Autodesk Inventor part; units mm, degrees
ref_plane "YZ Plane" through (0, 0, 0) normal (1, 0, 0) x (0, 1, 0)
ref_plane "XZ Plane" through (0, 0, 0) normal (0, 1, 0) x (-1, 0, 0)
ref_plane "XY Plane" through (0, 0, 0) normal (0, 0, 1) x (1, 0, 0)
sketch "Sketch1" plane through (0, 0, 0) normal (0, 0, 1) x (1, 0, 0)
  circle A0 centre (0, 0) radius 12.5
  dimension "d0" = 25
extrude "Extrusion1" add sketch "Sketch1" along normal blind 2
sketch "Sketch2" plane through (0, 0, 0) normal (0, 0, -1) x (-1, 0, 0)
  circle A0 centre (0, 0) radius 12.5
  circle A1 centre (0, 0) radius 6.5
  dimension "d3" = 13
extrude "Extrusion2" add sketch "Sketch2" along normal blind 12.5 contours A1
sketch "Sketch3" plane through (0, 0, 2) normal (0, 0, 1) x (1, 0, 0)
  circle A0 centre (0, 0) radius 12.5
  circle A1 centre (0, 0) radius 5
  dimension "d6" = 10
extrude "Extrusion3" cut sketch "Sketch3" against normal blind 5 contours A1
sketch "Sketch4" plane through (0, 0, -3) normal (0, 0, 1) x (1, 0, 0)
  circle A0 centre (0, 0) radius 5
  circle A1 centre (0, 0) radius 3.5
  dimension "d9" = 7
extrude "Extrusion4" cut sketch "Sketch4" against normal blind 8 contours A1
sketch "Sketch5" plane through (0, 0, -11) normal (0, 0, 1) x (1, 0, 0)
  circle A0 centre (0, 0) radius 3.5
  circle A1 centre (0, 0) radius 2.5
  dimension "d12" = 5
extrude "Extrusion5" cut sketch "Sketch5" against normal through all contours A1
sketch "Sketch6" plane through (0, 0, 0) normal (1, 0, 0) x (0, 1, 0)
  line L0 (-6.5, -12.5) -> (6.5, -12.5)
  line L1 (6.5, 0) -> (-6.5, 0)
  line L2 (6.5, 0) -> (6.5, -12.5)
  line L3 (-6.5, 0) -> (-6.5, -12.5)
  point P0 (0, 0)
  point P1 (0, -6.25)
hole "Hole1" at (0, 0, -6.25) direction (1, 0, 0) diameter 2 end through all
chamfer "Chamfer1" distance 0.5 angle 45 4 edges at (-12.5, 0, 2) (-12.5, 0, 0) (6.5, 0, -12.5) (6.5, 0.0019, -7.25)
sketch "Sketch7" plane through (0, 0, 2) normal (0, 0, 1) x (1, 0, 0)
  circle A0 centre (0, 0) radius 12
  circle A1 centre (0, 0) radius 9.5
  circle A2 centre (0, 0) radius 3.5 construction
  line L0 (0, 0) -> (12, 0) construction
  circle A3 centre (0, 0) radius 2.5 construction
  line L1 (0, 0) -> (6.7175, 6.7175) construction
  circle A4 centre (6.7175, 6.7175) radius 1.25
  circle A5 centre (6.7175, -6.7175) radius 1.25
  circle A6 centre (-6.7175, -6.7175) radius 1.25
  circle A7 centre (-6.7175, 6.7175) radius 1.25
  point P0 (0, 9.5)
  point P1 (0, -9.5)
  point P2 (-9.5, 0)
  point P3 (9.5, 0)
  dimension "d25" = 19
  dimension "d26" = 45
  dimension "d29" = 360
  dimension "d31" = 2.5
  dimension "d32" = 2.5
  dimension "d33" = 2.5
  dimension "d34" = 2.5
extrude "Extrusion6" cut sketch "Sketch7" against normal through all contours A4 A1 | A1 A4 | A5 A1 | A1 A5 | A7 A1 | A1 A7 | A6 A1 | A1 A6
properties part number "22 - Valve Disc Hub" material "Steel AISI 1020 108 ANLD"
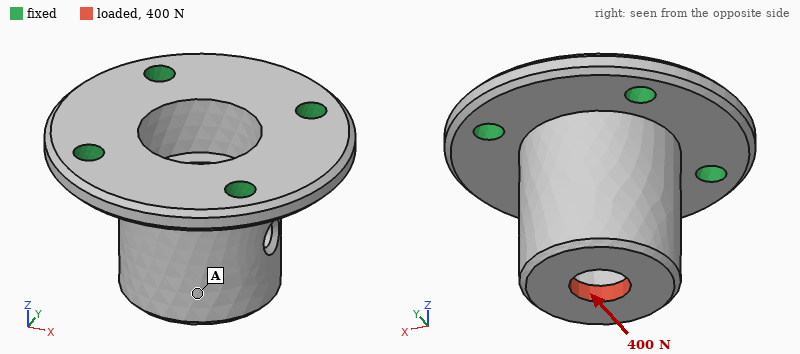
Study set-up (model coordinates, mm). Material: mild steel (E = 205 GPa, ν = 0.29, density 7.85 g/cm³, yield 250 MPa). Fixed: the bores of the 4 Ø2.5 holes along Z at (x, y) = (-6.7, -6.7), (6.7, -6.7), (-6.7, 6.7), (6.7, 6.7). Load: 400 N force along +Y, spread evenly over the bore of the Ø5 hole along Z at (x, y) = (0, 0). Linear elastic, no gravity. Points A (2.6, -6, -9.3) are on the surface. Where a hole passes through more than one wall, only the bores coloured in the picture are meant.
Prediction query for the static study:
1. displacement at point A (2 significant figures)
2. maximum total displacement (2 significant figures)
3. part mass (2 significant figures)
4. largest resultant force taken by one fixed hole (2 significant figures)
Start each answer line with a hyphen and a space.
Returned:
- 5.8 µm
- 7.4 µm
- 14 g
- 250 N
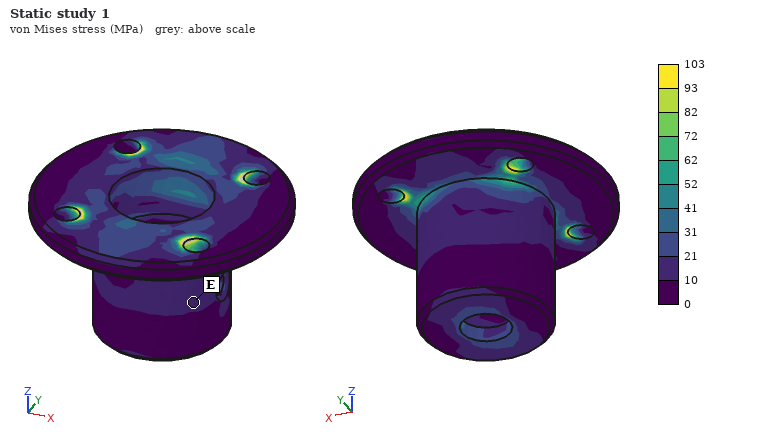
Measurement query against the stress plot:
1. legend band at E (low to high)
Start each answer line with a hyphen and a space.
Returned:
- 10 to 21 MPa
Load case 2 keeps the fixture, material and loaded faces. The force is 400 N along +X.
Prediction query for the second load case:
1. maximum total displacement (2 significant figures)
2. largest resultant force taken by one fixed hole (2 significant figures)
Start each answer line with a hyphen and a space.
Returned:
- 7.4 µm
- 250 N
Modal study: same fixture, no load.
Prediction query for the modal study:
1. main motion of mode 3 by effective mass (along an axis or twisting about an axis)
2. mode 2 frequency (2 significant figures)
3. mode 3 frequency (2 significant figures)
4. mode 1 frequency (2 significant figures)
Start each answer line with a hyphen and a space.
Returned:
- along Z
- 19 kHz
- 34 kHz
- 19 kHz
